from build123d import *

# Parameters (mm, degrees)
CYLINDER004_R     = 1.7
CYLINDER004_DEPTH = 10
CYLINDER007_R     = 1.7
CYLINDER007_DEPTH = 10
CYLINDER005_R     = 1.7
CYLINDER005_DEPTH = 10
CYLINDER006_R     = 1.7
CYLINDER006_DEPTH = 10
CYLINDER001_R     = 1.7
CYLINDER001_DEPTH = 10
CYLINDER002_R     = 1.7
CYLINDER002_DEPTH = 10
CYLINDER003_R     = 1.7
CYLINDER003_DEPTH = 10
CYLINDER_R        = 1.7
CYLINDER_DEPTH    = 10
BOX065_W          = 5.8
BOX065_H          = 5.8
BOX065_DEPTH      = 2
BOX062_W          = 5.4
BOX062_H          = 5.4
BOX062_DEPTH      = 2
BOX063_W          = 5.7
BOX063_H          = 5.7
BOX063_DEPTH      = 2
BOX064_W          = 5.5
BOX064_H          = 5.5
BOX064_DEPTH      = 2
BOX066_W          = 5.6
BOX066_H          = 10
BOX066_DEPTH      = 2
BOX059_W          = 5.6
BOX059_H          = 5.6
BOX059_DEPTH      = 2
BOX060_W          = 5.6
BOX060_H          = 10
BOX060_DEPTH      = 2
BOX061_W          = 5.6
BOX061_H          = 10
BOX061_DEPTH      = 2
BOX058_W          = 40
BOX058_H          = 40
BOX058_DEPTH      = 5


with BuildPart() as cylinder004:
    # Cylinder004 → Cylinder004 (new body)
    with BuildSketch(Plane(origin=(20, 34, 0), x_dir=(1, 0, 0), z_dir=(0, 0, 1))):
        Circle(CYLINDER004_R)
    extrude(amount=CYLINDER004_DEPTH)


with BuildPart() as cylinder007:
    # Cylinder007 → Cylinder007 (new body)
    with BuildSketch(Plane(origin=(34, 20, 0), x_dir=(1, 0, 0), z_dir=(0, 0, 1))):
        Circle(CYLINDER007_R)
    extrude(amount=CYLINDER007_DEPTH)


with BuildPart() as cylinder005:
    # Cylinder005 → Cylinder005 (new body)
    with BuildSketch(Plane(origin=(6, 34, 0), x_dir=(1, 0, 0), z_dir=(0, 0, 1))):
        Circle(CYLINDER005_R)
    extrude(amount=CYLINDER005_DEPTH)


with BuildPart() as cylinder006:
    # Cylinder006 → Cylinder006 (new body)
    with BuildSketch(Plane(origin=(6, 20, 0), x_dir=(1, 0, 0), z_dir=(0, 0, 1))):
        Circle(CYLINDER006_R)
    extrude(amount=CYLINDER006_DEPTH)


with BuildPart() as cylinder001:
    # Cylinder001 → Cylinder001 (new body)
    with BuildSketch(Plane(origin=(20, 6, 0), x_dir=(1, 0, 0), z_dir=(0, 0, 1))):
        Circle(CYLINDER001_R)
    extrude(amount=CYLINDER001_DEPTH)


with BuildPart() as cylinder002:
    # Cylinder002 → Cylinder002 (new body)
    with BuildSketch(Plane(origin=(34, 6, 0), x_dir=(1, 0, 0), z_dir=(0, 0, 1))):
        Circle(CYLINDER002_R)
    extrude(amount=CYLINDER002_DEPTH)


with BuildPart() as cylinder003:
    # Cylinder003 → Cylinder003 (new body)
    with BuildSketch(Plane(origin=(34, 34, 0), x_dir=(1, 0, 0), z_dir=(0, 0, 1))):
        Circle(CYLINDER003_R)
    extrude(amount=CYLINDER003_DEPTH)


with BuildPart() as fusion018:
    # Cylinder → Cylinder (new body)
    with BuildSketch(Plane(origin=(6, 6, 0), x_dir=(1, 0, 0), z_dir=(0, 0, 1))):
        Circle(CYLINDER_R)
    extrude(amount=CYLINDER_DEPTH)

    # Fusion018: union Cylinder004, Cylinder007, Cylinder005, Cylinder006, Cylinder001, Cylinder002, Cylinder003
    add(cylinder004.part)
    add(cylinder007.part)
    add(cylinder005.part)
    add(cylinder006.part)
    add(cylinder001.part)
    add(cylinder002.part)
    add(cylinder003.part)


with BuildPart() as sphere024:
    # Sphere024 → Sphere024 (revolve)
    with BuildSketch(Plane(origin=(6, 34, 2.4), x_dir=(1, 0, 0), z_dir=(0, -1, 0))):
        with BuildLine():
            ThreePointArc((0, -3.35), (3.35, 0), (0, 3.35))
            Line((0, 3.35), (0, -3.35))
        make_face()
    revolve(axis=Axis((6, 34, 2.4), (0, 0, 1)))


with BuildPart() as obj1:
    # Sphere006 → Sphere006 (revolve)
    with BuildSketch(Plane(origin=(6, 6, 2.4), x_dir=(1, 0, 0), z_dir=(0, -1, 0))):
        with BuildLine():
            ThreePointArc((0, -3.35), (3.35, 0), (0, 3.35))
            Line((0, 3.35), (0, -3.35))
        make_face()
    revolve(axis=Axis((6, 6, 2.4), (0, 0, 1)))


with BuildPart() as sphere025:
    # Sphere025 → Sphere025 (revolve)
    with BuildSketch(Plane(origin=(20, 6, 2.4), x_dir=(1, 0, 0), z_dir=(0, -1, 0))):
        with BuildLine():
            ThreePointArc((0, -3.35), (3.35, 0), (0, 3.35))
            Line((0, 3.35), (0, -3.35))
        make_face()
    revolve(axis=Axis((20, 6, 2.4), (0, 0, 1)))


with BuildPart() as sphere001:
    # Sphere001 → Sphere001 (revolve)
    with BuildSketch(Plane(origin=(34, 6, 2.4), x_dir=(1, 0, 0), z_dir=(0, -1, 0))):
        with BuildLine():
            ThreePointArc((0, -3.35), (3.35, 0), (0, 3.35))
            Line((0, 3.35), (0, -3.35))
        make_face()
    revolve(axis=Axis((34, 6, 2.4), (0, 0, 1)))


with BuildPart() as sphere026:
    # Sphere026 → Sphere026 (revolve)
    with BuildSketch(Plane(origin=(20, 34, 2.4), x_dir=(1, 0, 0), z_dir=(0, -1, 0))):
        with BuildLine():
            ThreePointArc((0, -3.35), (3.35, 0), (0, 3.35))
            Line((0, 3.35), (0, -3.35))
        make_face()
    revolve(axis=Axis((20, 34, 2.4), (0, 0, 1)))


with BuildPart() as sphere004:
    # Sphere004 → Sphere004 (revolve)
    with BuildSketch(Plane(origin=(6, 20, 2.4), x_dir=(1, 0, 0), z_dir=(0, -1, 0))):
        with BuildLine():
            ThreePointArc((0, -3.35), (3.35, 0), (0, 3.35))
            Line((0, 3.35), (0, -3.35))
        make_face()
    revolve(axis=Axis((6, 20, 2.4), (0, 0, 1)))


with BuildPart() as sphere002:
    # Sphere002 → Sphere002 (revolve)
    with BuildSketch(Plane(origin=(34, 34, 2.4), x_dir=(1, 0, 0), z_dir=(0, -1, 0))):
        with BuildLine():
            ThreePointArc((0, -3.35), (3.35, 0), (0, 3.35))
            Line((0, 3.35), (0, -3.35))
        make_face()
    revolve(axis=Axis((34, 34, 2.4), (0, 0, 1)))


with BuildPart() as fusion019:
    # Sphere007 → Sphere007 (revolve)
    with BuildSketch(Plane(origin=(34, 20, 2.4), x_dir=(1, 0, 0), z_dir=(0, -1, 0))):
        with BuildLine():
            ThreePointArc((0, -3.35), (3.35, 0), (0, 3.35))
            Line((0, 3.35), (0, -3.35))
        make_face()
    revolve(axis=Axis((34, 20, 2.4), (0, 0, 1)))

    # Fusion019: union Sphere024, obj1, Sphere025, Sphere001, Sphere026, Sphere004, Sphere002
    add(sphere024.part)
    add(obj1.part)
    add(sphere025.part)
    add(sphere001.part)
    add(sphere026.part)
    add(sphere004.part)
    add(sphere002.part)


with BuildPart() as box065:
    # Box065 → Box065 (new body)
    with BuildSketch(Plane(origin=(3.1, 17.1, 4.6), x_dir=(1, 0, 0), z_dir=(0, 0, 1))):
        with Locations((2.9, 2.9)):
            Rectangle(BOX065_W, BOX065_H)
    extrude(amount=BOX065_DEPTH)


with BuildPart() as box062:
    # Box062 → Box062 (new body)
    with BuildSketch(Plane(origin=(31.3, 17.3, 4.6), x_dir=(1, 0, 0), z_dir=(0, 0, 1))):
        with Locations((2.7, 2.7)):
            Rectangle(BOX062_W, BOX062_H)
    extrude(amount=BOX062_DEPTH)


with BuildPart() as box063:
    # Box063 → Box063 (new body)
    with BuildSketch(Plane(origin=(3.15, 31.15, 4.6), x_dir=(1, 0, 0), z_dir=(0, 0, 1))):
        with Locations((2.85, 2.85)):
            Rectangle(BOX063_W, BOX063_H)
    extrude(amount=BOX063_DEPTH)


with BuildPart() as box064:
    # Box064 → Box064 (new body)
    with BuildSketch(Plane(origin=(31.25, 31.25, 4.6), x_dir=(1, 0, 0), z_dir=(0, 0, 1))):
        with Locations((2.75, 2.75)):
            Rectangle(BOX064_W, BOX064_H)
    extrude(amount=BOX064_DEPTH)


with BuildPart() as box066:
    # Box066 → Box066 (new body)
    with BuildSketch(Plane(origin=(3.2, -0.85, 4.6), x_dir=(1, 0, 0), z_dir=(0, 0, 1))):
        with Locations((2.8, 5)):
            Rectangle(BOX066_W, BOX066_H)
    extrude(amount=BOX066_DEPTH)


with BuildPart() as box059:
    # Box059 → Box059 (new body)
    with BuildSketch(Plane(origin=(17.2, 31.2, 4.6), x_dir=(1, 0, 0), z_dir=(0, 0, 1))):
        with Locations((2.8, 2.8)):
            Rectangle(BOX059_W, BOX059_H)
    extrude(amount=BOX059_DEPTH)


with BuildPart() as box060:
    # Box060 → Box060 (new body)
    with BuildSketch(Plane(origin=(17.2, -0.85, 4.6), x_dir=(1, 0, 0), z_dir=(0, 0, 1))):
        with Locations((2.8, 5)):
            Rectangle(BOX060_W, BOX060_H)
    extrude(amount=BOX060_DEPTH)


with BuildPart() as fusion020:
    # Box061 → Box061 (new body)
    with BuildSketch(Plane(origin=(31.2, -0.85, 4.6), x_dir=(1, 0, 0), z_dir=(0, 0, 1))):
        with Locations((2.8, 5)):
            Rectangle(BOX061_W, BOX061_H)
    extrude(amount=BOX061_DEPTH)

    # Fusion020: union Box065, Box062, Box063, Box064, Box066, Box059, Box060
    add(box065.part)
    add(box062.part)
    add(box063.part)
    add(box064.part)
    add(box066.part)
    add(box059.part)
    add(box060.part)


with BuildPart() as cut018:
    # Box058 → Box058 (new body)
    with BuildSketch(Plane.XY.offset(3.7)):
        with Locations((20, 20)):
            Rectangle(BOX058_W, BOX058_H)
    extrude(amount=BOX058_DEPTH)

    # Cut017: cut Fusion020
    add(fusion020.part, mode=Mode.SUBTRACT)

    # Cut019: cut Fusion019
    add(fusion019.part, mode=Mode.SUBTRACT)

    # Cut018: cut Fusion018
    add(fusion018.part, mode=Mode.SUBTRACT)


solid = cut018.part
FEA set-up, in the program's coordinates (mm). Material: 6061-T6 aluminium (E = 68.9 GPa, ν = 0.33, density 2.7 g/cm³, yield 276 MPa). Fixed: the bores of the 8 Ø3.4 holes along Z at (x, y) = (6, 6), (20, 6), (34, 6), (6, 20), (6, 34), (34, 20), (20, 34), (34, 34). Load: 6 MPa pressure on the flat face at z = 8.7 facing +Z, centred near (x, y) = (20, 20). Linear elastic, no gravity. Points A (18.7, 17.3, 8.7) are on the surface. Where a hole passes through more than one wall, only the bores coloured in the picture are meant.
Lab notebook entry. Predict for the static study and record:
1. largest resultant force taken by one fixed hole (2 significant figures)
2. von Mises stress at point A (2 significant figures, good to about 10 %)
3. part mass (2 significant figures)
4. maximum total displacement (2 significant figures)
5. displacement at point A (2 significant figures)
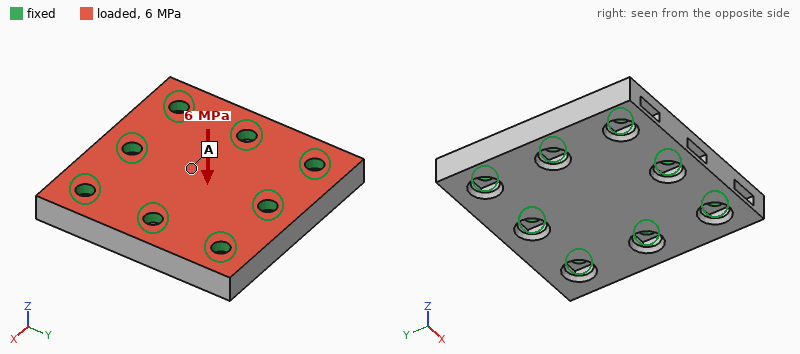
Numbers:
1.3 kN
21 MPa
19 g
14 µm
13 µm
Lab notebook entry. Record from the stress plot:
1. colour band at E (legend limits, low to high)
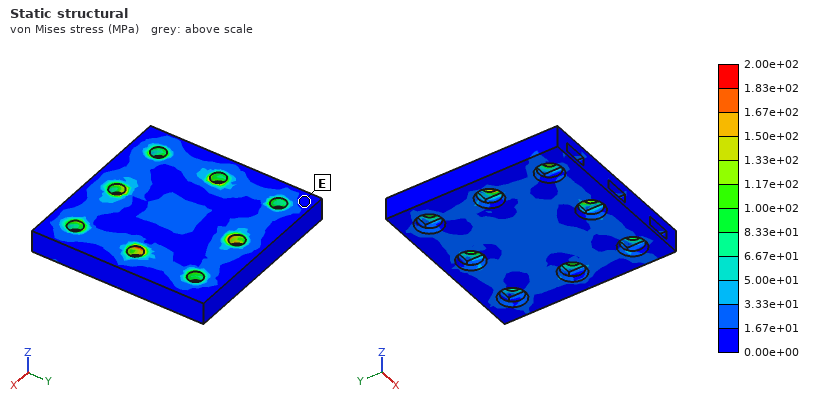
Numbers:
0.00e+00 to 1.67e+01 MPa
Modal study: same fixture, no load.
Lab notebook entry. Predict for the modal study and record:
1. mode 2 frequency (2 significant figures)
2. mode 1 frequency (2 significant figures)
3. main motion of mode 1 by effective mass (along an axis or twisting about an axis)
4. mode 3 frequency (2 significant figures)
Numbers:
45 kHz
33 kHz
along Z
46 kHz
